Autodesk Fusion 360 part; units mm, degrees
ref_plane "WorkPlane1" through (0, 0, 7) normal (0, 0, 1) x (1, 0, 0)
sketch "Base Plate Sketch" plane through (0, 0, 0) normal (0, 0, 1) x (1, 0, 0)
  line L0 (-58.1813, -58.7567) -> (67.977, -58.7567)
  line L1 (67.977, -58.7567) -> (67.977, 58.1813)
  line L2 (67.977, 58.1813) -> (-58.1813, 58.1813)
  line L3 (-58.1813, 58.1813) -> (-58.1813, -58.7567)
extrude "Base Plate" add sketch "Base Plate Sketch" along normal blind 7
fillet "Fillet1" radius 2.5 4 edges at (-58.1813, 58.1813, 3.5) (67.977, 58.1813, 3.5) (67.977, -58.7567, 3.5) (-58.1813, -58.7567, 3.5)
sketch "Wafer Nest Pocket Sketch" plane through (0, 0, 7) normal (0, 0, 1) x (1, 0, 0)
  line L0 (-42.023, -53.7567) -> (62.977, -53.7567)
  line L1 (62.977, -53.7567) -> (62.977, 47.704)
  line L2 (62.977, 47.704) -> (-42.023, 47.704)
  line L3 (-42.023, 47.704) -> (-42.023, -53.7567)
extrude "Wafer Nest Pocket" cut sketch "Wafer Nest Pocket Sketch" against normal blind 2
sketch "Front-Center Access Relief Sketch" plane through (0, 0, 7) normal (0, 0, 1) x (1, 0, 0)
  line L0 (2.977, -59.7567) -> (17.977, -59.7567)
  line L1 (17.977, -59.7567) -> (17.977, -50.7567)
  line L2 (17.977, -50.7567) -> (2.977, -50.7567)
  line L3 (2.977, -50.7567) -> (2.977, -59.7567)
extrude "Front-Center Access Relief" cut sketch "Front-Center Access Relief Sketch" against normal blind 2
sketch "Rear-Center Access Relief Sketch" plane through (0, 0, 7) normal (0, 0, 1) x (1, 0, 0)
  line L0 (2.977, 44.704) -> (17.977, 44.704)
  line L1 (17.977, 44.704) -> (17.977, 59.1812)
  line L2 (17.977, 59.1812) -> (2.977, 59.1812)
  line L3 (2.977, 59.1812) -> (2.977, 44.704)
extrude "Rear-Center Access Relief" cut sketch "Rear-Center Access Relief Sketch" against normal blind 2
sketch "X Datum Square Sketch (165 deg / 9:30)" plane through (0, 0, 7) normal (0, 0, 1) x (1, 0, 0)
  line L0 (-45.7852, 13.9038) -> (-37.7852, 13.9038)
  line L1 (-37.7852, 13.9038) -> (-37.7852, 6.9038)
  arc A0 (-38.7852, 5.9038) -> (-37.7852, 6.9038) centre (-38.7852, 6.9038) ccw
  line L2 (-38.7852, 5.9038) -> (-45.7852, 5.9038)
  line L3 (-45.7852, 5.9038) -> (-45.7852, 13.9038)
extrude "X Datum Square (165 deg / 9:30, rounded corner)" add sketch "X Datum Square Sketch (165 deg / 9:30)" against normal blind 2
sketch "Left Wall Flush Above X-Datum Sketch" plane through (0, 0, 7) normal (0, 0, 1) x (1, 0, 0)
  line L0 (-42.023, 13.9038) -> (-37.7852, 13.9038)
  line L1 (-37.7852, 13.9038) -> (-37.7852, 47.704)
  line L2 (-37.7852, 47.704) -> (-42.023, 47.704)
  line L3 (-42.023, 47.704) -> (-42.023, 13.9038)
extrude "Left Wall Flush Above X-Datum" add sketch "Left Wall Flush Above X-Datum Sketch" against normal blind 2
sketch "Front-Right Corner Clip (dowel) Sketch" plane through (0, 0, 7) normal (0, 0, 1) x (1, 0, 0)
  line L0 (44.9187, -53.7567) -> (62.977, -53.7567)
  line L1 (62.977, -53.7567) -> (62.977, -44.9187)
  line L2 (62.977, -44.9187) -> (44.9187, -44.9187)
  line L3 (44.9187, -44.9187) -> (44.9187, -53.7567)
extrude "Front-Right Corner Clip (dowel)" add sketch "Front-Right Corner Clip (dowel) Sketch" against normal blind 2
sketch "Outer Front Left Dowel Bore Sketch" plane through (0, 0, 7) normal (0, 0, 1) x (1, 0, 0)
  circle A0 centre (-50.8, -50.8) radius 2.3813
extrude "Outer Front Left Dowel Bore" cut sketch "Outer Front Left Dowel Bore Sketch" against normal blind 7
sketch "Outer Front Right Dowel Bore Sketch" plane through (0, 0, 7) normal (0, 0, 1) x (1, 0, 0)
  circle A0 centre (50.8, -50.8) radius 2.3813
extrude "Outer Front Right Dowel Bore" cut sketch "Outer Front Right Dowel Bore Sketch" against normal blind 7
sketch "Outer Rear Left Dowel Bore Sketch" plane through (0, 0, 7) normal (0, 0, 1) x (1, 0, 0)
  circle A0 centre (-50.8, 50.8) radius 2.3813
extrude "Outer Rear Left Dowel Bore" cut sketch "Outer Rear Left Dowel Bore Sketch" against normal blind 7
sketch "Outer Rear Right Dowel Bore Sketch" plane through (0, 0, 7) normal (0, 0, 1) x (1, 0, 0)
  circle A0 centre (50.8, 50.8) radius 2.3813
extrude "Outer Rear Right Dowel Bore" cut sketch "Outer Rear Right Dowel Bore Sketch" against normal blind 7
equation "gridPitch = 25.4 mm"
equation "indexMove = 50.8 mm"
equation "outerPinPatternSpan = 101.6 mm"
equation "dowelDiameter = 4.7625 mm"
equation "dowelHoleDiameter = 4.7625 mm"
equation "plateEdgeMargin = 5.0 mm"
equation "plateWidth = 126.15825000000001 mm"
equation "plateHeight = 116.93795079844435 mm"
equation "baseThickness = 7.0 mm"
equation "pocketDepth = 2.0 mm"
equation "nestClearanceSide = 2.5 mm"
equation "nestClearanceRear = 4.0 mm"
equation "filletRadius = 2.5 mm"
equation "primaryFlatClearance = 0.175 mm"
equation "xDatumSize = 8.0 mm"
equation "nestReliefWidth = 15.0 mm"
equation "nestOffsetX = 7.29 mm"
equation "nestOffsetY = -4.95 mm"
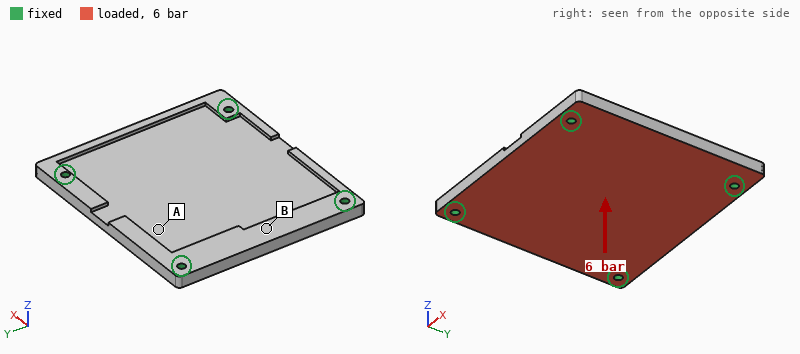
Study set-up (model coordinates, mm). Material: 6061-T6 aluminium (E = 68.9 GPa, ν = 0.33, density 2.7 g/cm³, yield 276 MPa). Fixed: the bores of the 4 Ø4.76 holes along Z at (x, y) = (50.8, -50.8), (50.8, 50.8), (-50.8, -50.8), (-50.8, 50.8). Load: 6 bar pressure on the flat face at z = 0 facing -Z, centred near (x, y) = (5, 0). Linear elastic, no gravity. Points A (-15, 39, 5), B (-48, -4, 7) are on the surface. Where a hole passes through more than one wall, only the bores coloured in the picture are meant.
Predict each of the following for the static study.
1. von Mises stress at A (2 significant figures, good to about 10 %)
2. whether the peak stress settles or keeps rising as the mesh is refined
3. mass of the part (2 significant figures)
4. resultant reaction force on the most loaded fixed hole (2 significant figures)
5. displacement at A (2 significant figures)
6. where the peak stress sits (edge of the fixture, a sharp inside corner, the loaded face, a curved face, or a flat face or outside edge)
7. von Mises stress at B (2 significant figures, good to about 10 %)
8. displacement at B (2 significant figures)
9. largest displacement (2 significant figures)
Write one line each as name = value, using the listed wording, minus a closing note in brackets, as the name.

von Mises stress at A = 31 MPa
whether the peak stress settles or keeps rising as the mesh is refined = keeps rising
mass of the part = 220 g
resultant reaction force on the most loaded fixed hole = 2.7 kN
displacement at A = 0.24 mm
where the peak stress sits = edge of the fixture
von Mises stress at B = 68 MPa
displacement at B = 0.20 mm
largest displacement = 0.47 mm
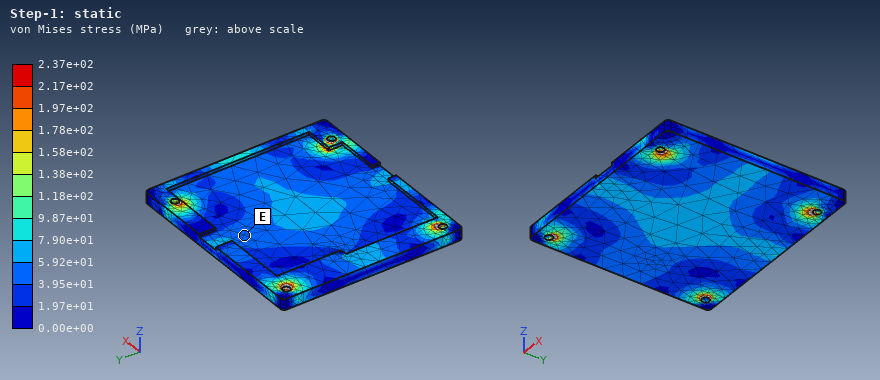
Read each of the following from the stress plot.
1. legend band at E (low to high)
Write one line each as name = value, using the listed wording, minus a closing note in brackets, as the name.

legend band at E = 3.95e+01 to 5.92e+01 MPa
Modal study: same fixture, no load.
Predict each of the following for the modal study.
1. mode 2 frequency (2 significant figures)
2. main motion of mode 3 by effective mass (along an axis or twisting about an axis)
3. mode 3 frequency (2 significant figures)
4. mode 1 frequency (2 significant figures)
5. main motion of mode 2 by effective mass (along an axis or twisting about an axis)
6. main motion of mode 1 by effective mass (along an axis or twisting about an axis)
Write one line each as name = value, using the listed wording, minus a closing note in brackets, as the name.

mode 2 frequency = 3000 Hz
main motion of mode 3 by effective mass = twisting about X
mode 3 frequency = 3200 Hz
mode 1 frequency = 1900 Hz
main motion of mode 2 by effective mass = twisting about Y
main motion of mode 1 by effective mass = along Z
